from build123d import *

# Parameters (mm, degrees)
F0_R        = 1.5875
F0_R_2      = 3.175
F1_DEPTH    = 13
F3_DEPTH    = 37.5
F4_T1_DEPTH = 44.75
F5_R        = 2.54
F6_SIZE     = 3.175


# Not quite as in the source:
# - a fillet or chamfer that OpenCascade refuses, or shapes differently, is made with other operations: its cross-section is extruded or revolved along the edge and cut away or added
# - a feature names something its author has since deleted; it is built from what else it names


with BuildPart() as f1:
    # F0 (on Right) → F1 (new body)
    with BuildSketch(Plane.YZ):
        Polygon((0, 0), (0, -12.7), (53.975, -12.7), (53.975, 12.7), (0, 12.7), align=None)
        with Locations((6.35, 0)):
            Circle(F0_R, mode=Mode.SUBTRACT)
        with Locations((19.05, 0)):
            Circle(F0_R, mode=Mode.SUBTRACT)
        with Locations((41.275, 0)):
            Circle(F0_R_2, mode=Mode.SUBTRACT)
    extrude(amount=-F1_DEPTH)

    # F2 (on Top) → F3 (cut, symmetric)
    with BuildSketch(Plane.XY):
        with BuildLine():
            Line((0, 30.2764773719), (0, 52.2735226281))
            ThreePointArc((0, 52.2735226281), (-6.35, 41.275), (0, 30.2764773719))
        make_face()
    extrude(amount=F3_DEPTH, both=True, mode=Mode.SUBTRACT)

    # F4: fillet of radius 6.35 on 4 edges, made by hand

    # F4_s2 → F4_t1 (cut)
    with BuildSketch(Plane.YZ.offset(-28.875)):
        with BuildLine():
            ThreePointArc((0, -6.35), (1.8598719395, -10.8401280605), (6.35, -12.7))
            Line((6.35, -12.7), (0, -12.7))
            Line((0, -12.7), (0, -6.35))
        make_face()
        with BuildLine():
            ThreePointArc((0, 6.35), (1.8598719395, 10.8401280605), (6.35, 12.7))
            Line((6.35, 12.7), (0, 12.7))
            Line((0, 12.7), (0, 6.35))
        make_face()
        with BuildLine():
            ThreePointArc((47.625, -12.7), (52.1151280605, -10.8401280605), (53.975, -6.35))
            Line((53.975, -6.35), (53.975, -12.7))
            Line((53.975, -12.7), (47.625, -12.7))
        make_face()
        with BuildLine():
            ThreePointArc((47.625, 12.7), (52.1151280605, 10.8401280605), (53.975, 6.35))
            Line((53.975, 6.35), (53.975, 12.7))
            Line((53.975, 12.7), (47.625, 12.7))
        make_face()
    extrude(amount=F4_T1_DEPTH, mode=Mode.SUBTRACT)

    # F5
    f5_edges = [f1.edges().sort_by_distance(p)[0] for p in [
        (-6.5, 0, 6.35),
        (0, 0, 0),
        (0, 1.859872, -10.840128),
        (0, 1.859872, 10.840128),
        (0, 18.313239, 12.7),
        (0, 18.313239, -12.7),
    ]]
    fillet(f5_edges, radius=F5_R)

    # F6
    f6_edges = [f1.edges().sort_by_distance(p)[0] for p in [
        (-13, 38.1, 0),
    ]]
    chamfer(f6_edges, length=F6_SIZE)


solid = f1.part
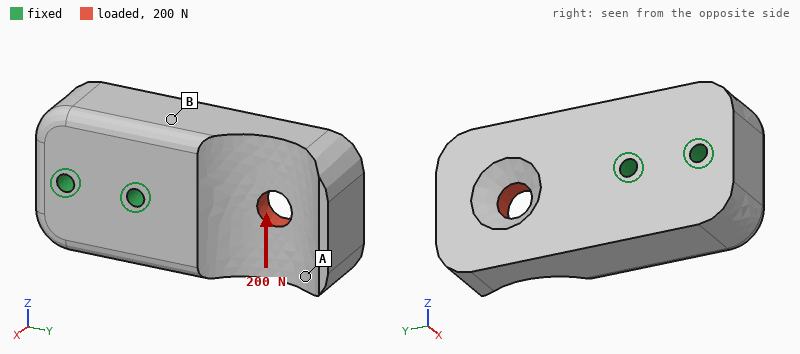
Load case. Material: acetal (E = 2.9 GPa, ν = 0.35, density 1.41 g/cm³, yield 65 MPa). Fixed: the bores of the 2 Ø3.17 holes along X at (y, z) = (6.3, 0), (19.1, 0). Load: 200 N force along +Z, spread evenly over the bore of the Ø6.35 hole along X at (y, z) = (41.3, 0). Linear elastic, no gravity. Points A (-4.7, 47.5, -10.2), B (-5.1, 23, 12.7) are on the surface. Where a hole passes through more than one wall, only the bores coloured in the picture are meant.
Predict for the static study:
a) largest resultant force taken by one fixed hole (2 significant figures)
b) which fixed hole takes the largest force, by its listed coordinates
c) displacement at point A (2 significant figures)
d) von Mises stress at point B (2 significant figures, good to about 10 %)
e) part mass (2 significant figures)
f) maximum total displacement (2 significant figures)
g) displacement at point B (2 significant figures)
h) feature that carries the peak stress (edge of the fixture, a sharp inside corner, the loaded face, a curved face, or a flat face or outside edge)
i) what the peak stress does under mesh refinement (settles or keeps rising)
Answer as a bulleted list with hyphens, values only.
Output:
- 470 N
- (19.1, 0)
- 0.10 mm
- 3.1 MPa
- 20 g
- 0.12 mm
- 0.027 mm
- edge of the fixture
- keeps rising
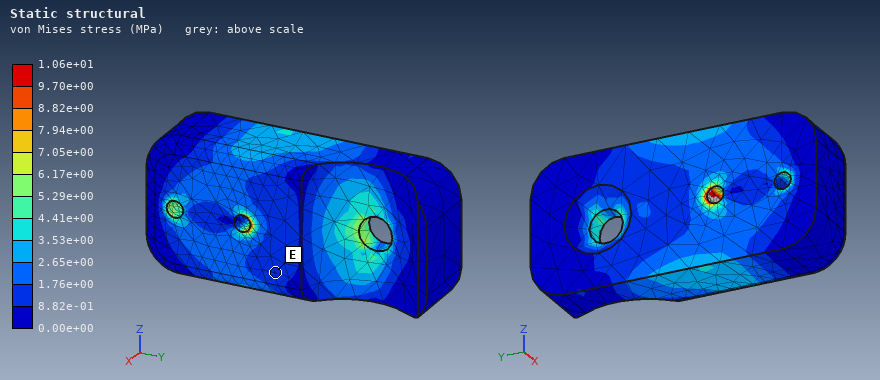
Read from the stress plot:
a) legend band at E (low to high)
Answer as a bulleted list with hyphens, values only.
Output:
- 8.82e-01 to 1.76e+00 MPa
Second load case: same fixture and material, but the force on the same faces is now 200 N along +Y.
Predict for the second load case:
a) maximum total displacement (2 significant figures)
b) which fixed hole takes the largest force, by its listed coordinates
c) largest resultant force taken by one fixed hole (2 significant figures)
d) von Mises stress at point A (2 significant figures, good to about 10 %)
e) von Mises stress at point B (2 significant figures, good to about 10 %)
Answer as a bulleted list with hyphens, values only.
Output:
- 22 µm
- (19.1, 0)
- 150 N
- 0.58 MPa
- 0.36 MPa
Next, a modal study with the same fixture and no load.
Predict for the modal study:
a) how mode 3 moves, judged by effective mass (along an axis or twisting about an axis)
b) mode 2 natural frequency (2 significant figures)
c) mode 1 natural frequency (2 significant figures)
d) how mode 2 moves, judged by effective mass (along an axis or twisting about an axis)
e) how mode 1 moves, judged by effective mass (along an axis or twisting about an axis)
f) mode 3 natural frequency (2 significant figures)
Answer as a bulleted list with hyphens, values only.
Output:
- twisting about Y
- 2700 Hz
- 1900 Hz
- along Z
- along X
- 4200 Hz
